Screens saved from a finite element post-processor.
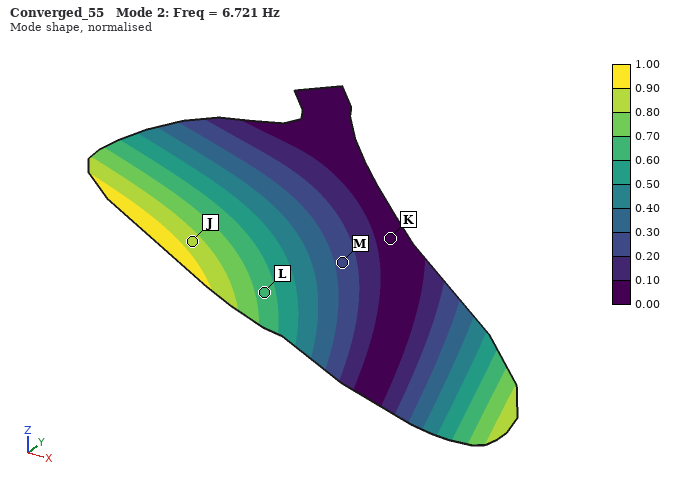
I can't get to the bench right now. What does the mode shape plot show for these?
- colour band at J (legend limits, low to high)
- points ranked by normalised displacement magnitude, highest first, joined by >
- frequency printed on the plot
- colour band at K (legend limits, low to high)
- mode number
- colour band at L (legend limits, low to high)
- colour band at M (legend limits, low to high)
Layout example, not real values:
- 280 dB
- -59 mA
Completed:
- 0.80 to 0.90
- J > L > M > K
- 6.721 Hz
- 0.00 to 0.10
- 2
- 0.60 to 0.70
- 0.20 to 0.30
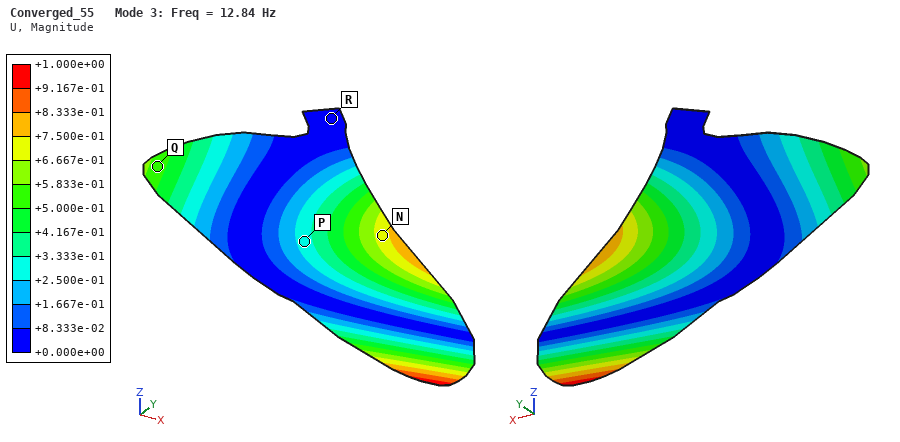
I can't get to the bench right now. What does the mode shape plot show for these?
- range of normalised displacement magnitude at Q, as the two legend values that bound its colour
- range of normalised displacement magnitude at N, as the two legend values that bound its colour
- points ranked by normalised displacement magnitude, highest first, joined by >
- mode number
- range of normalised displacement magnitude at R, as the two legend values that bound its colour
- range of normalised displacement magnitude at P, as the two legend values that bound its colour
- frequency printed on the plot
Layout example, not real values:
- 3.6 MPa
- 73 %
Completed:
- +5.000e-01 to +5.833e-01
- +6.667e-01 to +7.500e-01
- N > Q > P > R
- 3
- +0.000e+00 to +8.333e-02
- +2.500e-01 to +3.333e-01
- 12.84 Hz
